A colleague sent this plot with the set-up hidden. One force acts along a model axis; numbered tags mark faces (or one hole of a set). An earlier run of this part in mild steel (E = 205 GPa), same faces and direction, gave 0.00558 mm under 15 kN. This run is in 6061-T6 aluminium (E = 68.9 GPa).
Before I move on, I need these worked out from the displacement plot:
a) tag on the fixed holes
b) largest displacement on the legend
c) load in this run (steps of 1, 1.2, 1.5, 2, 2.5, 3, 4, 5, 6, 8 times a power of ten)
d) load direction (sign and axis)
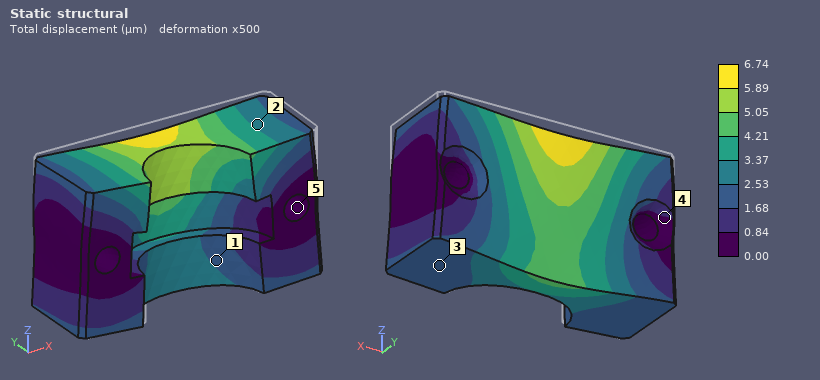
5
6.74 µm
6 kN
-Z
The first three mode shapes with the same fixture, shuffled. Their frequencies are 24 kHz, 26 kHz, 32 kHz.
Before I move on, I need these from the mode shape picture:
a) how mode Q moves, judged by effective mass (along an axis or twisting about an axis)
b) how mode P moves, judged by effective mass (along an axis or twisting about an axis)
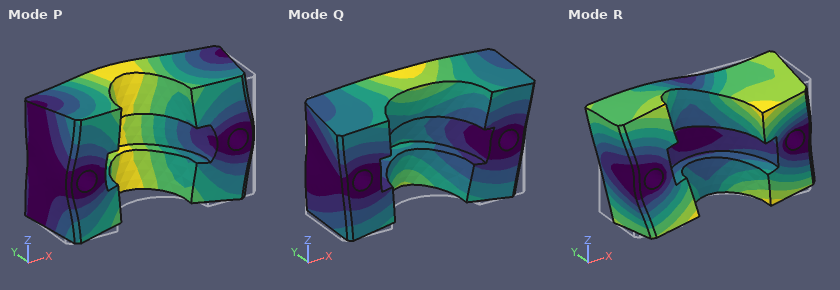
along Z
along Y
